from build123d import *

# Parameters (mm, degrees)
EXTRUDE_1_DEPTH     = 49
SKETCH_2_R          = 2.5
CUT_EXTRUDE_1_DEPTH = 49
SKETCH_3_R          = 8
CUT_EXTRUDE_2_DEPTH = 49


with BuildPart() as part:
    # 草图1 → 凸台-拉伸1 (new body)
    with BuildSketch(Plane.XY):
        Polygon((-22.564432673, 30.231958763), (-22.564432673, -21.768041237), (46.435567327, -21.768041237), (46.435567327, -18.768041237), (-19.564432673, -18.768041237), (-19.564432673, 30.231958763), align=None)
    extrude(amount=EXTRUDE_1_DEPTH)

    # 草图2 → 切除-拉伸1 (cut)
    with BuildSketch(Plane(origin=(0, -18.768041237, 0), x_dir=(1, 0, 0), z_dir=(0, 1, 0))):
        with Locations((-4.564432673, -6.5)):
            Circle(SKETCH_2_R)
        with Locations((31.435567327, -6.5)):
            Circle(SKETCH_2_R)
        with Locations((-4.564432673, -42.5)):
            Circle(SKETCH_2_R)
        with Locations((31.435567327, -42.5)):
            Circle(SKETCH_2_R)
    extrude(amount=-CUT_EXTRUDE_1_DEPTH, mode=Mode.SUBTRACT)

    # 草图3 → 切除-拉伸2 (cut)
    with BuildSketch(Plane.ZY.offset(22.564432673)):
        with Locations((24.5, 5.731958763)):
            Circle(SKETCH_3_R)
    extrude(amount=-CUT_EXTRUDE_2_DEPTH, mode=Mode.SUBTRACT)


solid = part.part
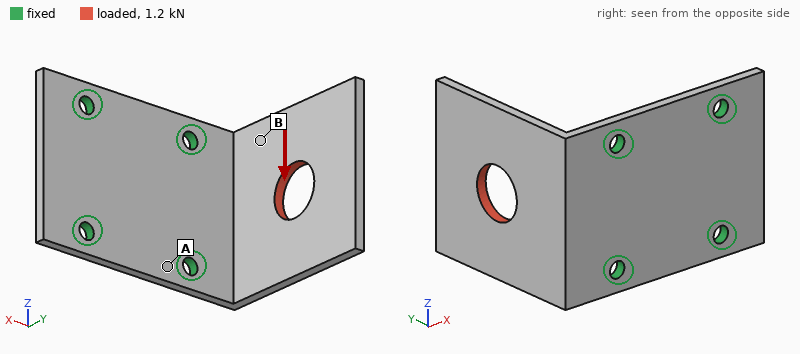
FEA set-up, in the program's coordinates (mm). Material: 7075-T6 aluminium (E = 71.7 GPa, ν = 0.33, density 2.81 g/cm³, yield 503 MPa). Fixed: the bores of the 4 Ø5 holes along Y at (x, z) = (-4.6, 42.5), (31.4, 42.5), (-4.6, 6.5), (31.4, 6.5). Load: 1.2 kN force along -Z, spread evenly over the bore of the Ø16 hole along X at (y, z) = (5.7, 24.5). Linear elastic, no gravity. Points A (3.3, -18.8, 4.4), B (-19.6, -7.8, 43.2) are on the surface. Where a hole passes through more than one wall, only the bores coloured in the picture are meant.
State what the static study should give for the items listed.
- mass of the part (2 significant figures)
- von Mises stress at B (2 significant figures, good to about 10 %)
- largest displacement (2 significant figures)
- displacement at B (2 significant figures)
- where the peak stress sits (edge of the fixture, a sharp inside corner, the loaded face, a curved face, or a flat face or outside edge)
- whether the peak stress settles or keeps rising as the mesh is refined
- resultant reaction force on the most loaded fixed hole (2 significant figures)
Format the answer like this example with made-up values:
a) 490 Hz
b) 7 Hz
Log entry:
a) 46 g
b) 68 MPa
c) 0.62 mm
d) 0.24 mm
e) edge of the fixture
f) keeps rising
g) 1.1 kN
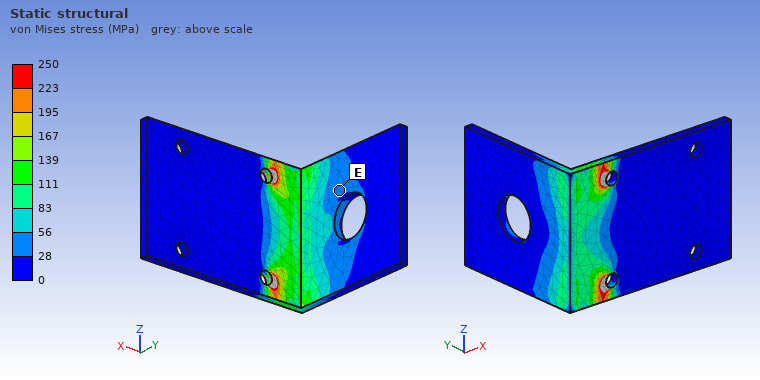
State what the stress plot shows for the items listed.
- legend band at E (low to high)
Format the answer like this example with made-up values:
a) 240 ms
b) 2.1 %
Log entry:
a) 28 to 56 MPa
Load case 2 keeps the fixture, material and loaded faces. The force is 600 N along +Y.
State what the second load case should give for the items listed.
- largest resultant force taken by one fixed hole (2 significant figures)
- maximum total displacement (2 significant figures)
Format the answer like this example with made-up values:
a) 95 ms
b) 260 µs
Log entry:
a) 320 N
b) 0.50 mm
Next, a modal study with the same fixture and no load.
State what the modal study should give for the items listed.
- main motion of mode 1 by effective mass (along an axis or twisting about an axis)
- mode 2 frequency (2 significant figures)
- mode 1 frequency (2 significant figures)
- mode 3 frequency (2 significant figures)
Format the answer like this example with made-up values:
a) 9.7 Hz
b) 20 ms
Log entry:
a) along X
b) 1700 Hz
c) 660 Hz
d) 2400 Hz
